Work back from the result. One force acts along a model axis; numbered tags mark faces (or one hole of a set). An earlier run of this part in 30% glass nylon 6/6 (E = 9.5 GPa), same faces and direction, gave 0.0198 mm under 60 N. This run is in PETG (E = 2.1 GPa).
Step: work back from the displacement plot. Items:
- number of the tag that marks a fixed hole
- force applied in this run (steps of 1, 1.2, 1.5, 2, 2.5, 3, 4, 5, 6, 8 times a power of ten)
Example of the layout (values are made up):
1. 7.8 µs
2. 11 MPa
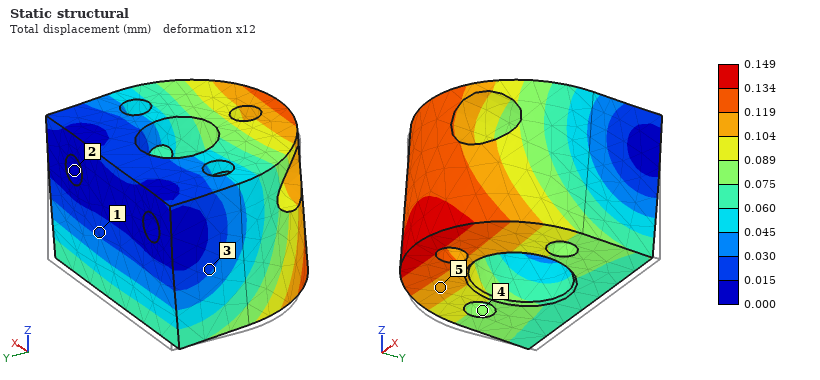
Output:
1. 2
2. 100 N
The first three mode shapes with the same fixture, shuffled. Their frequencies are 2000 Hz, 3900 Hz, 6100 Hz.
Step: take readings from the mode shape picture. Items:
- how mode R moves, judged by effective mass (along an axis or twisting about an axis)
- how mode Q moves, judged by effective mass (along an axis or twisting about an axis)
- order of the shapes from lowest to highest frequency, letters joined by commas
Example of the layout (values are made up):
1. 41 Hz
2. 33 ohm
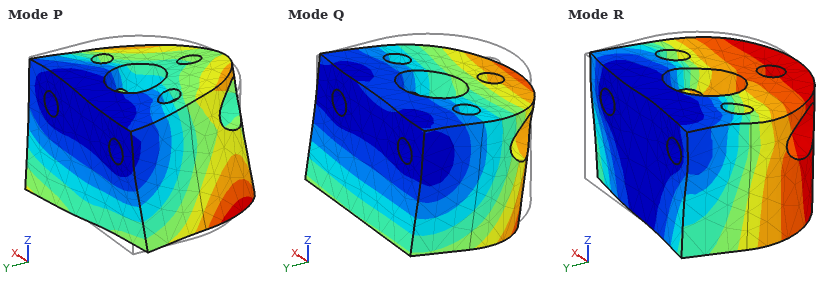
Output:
1. along X
2. along Z
3. Q, R, P
